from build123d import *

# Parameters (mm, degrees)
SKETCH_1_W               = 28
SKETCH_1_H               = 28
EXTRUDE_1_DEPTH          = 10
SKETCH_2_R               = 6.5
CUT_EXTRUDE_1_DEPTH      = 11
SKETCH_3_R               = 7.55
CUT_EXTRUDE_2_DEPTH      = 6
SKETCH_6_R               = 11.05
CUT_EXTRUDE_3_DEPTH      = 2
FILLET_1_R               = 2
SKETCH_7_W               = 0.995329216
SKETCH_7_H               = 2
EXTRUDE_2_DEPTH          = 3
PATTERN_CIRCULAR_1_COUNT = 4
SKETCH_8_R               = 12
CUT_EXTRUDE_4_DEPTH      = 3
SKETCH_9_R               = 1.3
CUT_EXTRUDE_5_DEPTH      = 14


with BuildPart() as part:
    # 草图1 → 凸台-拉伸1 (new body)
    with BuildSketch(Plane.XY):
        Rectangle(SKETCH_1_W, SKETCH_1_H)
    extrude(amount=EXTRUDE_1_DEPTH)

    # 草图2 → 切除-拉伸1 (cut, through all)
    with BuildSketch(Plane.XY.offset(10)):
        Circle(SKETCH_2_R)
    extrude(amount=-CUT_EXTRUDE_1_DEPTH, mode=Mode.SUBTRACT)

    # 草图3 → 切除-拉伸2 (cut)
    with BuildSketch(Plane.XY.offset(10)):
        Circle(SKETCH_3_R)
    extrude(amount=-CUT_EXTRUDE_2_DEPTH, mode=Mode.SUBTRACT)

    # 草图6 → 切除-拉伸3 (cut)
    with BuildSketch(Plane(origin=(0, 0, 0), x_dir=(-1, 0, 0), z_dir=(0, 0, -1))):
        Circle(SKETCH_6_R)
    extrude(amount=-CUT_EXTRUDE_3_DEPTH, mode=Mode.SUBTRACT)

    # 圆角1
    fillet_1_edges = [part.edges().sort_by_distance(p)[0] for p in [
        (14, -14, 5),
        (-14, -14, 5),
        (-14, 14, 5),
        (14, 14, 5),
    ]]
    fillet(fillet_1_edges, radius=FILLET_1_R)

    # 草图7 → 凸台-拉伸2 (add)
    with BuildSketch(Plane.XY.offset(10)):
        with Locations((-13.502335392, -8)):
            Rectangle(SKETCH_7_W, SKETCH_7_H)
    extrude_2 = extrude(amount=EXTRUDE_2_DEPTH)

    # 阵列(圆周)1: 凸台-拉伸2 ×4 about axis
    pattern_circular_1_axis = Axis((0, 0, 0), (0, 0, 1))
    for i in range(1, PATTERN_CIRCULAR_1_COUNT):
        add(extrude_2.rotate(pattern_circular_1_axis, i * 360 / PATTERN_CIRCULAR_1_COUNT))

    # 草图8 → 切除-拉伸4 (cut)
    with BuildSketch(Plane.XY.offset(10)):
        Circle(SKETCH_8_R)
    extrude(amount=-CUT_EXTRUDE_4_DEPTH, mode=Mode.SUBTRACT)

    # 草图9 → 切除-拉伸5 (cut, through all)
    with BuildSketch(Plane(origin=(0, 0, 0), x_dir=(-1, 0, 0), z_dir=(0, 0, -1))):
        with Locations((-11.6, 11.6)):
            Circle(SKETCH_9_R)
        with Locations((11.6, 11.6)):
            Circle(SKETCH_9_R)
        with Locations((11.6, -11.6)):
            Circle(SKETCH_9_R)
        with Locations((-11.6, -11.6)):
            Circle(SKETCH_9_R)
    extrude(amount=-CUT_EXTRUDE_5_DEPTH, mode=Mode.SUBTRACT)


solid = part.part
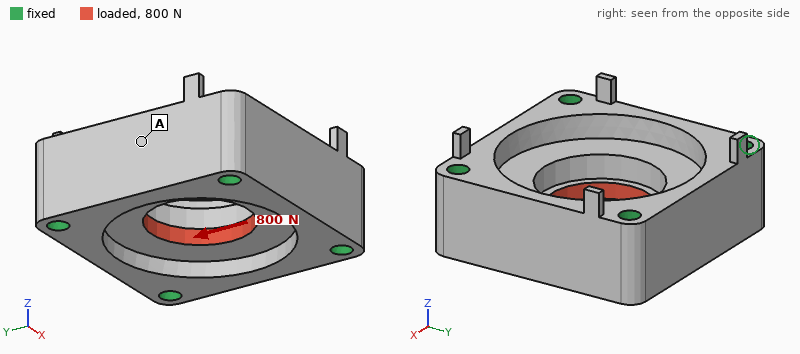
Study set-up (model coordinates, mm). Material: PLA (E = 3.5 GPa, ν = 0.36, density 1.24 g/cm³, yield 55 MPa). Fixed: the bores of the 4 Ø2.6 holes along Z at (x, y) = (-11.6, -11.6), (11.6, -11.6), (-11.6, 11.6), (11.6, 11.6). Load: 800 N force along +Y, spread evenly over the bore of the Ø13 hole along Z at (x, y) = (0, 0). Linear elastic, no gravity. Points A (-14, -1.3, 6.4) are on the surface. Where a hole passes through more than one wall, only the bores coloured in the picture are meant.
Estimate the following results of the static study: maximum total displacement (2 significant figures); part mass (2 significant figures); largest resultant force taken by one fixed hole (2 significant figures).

40 µm
5.8 g
210 N
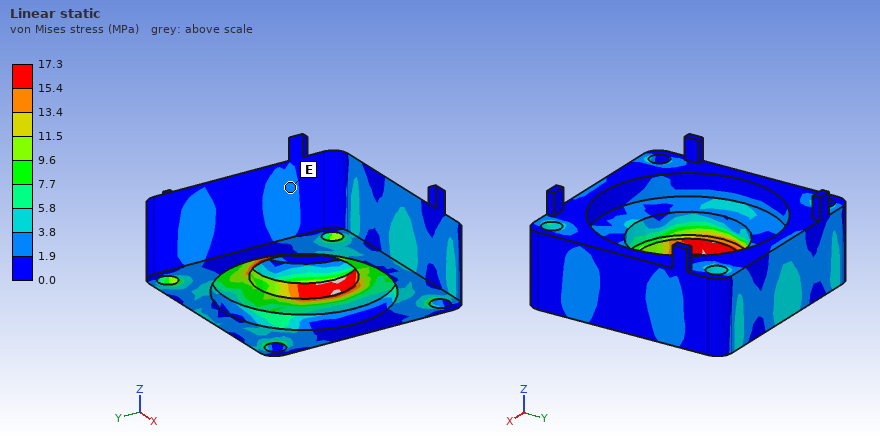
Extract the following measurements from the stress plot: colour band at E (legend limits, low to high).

1.9 to 3.8 MPa
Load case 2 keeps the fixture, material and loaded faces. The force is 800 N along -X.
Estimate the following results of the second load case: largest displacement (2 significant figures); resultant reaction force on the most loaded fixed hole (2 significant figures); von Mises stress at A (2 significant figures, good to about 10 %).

41 µm
210 N
4.0 MPa
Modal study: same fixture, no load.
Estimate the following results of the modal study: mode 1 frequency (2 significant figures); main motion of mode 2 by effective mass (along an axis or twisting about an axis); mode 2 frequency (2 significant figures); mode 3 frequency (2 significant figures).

13 kHz
along Z
17 kHz
19 kHz
